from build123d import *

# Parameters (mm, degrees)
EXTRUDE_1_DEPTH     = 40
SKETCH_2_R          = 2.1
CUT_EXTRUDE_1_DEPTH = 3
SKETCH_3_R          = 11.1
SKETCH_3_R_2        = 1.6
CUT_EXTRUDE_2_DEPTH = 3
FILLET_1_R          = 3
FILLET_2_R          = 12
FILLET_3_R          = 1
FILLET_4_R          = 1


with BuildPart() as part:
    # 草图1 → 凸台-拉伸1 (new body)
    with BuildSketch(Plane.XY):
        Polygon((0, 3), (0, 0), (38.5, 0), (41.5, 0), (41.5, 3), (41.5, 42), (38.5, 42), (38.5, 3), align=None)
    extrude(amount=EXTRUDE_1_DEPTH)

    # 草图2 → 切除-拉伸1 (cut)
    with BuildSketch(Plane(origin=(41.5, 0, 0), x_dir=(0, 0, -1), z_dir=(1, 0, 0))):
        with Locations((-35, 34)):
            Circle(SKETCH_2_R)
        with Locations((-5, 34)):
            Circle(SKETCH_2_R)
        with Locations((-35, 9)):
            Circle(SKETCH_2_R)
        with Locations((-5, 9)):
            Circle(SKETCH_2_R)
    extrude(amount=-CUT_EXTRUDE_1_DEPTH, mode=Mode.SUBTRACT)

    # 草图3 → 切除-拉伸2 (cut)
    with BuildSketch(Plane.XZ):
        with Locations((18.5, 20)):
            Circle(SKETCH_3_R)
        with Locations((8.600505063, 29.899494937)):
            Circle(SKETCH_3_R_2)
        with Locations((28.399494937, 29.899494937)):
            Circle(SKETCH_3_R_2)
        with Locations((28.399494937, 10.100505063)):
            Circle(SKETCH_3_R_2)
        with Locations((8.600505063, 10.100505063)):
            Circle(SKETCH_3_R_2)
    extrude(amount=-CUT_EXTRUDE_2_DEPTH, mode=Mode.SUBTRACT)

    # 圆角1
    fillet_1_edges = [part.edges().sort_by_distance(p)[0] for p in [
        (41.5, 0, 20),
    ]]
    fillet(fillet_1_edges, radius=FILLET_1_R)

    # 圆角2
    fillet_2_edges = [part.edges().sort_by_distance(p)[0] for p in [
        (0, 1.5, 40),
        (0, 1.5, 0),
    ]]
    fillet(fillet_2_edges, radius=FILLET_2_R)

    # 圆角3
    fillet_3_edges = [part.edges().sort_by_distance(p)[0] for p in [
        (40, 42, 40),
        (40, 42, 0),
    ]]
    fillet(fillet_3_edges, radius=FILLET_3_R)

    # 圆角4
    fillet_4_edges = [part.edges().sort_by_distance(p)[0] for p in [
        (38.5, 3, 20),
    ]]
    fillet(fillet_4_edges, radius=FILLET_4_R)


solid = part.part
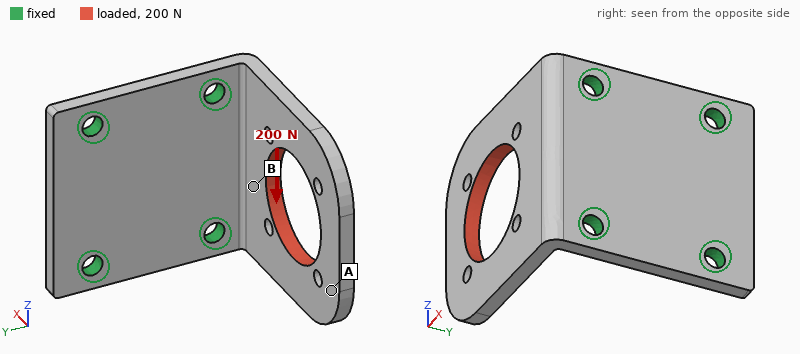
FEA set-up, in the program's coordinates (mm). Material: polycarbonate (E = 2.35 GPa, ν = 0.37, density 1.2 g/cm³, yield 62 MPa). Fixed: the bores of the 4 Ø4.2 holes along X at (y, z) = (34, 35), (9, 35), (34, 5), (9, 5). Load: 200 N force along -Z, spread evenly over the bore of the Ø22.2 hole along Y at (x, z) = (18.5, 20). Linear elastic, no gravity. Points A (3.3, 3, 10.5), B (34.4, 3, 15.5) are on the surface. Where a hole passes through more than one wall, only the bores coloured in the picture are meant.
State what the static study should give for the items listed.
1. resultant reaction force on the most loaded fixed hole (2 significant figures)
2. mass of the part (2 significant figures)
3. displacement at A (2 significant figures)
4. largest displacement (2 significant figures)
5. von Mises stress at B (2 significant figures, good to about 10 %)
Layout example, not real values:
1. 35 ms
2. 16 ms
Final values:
1. 170 N
2. 9.6 g
3. 0.69 mm
4. 0.76 mm
5. 11 MPa
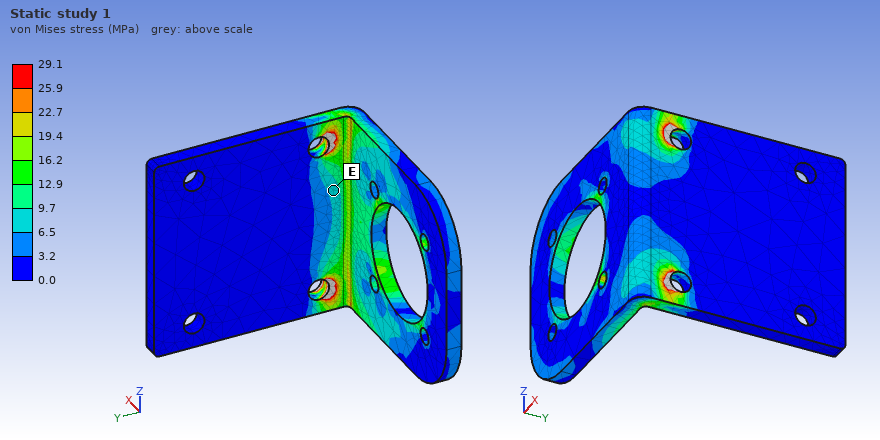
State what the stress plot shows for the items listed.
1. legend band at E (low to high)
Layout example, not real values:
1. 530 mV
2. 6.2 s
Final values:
1. 6.5 to 9.7 MPa
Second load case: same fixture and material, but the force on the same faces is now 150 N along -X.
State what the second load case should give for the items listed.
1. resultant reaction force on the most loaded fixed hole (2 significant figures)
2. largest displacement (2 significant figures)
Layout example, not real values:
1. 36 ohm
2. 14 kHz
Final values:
1. 79 N
2. 0.73 mm
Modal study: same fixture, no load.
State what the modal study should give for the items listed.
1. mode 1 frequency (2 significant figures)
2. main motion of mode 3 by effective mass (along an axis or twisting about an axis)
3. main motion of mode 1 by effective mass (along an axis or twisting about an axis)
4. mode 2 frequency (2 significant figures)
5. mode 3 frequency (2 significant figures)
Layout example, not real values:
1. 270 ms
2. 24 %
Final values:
1. 370 Hz
2. along Z
3. along Y
4. 880 Hz
5. 1700 Hz
